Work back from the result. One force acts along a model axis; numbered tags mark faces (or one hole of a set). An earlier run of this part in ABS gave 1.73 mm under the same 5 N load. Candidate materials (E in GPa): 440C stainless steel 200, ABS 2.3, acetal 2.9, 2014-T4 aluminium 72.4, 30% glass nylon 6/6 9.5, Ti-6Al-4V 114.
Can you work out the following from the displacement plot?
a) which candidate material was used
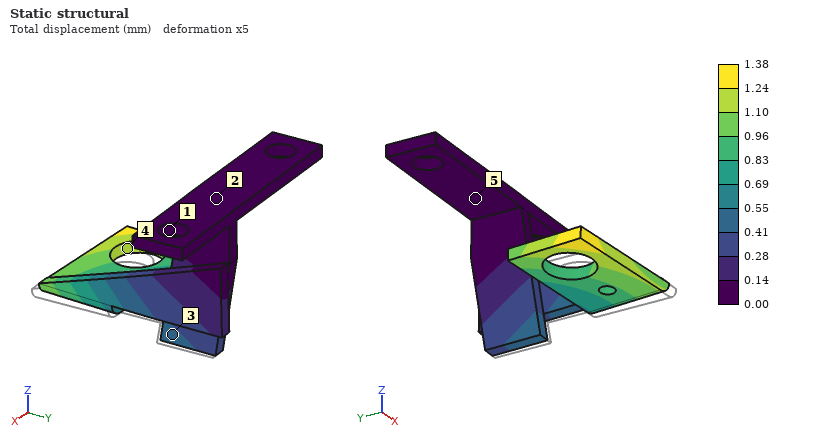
acetal
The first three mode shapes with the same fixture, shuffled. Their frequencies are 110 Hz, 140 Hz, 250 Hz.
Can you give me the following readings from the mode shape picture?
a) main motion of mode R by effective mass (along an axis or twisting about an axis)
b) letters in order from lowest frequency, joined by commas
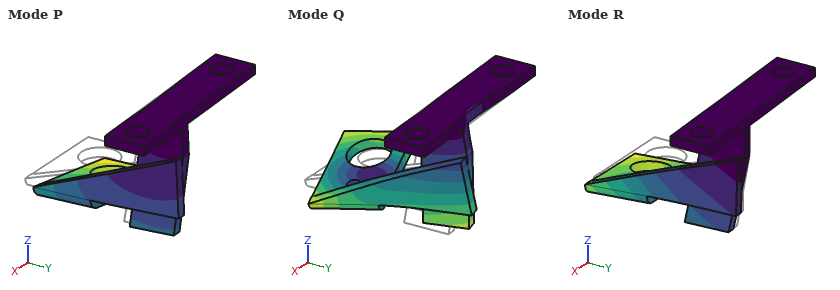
along X
R, P, Q
